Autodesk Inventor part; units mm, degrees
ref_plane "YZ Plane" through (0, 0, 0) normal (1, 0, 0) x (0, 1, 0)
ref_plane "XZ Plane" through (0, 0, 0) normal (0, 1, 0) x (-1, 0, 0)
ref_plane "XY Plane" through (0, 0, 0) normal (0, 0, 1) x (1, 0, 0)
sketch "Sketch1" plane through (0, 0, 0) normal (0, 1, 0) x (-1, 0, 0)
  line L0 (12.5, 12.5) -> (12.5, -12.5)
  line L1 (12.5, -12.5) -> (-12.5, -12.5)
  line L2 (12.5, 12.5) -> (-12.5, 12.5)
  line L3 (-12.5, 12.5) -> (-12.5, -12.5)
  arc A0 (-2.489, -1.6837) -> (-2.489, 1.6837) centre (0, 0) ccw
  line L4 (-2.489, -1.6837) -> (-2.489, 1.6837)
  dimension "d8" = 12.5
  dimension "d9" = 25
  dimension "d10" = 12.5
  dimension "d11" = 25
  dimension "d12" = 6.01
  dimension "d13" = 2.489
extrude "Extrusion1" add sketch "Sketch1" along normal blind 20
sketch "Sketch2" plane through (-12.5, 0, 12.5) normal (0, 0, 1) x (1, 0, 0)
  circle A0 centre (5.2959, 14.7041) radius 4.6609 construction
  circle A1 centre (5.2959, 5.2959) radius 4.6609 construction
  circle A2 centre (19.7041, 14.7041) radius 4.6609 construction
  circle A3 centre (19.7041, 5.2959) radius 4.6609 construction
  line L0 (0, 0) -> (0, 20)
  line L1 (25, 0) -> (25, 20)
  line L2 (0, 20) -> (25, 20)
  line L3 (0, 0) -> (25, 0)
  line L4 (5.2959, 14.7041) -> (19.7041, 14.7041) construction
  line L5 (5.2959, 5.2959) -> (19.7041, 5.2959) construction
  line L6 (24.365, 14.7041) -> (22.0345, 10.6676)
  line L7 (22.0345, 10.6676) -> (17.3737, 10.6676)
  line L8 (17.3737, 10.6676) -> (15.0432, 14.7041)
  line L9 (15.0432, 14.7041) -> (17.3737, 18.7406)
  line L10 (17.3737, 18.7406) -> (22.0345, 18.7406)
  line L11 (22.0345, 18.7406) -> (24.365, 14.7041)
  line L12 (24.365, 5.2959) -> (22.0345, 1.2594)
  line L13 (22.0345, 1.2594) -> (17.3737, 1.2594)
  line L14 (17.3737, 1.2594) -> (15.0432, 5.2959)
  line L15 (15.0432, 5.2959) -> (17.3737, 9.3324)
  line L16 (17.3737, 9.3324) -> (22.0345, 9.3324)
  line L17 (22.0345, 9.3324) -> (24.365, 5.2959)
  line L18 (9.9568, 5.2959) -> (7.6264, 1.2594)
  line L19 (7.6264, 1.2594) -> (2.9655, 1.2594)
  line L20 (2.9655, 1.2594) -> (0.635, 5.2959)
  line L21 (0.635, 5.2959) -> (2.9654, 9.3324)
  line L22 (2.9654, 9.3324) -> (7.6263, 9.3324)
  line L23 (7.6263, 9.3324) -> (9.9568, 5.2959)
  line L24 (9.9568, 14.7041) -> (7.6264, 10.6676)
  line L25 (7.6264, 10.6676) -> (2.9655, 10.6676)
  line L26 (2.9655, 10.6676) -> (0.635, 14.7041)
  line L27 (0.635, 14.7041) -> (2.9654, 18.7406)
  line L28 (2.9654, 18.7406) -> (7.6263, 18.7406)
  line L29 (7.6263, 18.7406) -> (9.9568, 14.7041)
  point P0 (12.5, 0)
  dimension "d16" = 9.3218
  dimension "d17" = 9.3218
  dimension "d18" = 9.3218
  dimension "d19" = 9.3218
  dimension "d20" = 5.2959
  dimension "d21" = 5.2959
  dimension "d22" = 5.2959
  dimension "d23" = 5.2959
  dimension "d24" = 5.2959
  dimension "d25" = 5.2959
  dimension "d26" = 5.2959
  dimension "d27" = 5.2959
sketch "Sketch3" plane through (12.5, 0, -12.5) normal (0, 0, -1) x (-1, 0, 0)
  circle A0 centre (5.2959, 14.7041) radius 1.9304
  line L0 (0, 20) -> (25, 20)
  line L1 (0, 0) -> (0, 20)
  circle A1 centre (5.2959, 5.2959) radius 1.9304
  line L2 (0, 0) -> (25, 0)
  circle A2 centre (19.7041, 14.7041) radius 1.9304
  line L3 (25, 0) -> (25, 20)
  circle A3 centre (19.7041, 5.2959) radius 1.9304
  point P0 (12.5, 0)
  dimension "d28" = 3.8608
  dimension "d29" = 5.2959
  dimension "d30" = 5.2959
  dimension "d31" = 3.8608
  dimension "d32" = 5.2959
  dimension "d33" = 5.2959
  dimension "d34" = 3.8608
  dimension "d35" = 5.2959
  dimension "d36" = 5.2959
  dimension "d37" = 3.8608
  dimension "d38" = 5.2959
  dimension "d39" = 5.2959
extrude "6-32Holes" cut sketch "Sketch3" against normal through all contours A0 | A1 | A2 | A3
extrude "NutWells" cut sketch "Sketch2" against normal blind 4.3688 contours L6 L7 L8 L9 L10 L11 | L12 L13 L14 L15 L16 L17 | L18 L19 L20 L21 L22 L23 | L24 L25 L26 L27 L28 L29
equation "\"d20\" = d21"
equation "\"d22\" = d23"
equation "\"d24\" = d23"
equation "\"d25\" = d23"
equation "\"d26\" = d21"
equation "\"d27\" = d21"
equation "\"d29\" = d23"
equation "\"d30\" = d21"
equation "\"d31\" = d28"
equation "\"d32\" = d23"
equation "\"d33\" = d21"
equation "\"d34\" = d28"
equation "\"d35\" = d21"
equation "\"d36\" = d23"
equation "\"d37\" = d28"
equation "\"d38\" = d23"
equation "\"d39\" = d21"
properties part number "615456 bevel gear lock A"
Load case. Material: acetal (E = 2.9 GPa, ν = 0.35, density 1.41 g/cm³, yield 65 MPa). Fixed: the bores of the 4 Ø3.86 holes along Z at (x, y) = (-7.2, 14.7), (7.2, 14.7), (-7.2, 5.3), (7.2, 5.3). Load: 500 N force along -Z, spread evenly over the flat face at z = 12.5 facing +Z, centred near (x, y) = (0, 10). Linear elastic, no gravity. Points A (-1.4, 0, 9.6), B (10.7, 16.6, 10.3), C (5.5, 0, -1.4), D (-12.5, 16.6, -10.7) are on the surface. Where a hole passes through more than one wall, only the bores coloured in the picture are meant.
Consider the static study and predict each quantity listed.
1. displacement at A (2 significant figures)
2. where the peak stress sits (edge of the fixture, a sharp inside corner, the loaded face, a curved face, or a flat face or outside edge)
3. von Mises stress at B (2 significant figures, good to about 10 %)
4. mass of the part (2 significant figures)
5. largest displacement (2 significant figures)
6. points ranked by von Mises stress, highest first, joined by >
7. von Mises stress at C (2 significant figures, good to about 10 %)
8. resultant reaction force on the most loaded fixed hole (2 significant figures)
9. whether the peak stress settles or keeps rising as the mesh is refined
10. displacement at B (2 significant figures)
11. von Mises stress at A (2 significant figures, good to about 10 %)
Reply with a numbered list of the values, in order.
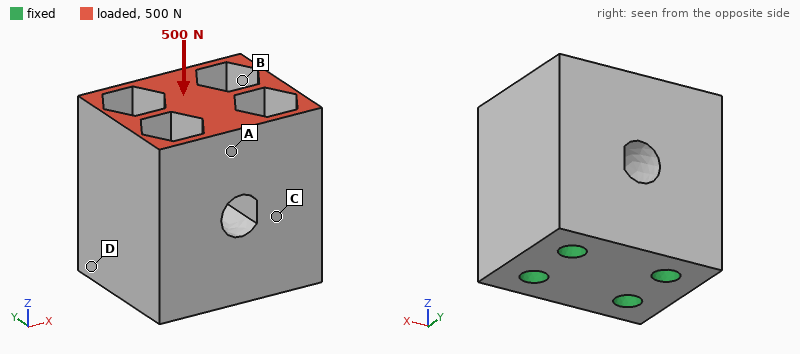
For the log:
1. 6.5 µm
2. edge of the fixture
3. 2.1 MPa
4. 14 g
5. 8.2 µm
6. B > A > C > D
7. 0.56 MPa
8. 130 N
9. keeps rising
10. 4.8 µm
11. 1.3 MPa
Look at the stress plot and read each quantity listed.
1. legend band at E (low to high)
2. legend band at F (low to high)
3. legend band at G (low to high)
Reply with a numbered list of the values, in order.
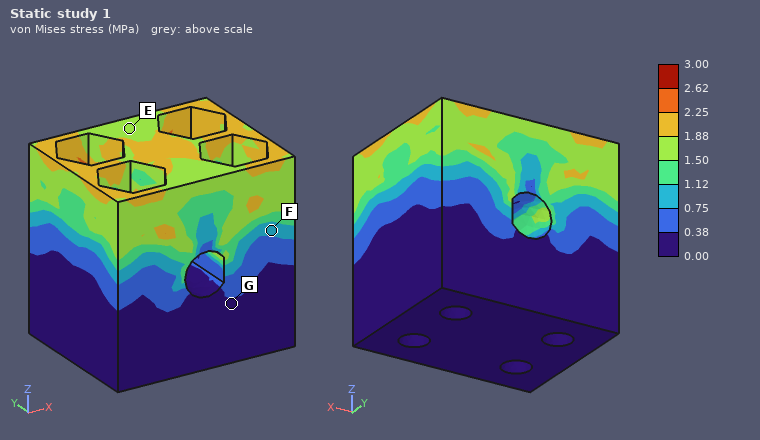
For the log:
1. 1.50 to 1.88 MPa
2. 0.75 to 1.12 MPa
3. 0.00 to 0.38 MPa
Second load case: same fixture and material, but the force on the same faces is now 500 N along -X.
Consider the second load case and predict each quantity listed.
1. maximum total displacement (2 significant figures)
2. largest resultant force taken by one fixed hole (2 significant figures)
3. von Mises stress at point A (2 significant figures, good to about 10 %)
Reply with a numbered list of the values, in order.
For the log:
1. 41 µm
2. 160 N
3. 4.3 MPa
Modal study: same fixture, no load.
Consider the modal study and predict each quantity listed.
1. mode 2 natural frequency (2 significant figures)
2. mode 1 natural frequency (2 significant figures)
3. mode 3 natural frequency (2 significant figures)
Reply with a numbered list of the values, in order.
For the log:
1. 24 kHz
2. 20 kHz
3. 24 kHz
